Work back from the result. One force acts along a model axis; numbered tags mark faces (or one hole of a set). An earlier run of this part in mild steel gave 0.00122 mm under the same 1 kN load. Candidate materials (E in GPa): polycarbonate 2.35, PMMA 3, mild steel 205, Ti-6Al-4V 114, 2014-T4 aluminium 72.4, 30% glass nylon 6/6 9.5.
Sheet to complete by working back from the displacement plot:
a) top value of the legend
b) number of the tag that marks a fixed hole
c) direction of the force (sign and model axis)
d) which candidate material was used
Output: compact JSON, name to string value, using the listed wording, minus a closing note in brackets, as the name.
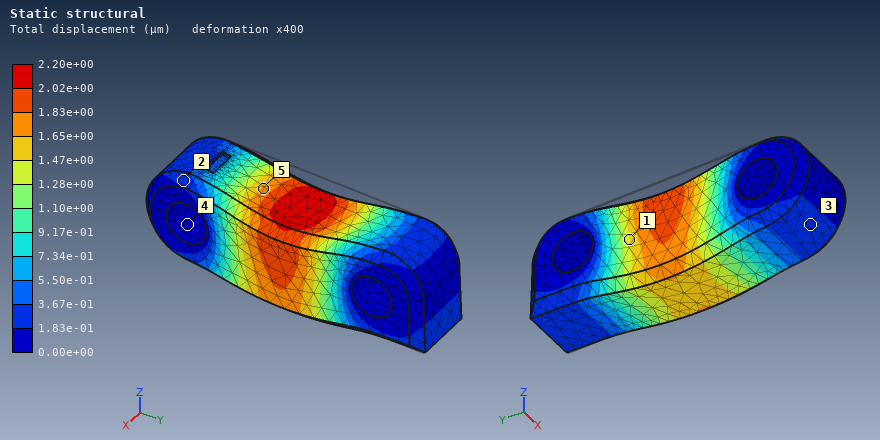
{"top value of the legend": "2.20e+00 µm", "number of the tag that marks a fixed hole": "4", "direction of the force": "-Z", "which candidate material was used": "Ti-6Al-4V"}
